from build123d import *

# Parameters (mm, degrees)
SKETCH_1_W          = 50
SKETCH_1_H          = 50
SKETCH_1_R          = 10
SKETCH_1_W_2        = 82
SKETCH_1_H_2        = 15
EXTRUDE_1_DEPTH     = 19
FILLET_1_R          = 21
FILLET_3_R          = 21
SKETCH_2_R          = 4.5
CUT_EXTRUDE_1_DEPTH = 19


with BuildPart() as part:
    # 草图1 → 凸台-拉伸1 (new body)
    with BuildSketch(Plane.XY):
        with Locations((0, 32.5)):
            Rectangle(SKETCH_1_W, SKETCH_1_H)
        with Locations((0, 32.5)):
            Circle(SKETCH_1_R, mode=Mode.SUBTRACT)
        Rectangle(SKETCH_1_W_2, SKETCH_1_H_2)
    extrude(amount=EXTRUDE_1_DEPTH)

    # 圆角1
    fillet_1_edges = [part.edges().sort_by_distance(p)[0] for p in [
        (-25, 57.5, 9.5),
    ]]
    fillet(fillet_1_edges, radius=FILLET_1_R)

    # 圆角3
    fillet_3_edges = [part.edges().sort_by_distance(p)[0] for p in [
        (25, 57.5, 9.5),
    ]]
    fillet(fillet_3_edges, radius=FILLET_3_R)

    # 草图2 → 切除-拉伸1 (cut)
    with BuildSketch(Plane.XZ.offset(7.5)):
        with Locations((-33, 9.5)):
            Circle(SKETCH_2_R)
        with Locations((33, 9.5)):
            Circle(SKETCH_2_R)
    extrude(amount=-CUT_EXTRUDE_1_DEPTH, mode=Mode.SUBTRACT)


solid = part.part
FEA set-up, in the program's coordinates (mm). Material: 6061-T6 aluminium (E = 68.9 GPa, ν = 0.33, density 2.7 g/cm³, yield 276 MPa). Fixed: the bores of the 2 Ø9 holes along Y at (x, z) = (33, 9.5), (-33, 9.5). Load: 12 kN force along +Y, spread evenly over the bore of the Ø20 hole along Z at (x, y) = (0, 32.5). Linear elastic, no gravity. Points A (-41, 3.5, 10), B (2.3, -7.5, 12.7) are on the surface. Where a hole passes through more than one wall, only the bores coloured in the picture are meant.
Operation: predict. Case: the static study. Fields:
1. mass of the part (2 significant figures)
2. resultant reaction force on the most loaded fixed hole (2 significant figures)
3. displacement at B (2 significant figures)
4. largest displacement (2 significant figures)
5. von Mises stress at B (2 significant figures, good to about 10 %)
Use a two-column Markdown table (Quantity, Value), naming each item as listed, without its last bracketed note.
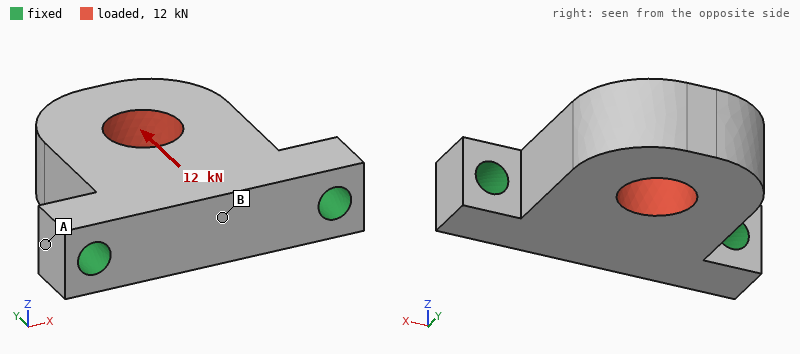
| Quantity | Value |
|---|---|
| mass of the part | 160 g |
| resultant reaction force on the most loaded fixed hole | 6.4 kN |
| displacement at B | 16 µm |
| largest displacement | 23 µm |
| von Mises stress at B | 15 MPa |
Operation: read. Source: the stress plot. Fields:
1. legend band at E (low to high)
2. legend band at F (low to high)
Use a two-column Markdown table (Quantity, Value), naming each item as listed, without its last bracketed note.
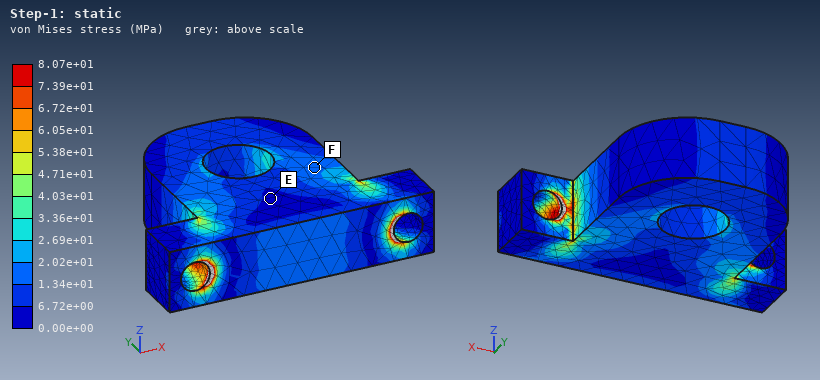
| Quantity | Value |
|---|---|
| legend band at E | 0.00e+00 to 6.72e+00 MPa |
| legend band at F | 1.34e+01 to 2.02e+01 MPa |
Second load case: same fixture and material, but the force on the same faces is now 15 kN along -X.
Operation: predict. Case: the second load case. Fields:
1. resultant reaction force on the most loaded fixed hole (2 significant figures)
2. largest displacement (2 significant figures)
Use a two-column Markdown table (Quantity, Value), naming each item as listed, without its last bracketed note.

| Quantity | Value |
|---|---|
| resultant reaction force on the most loaded fixed hole | 11 kN |
| largest displacement | 84 µm |
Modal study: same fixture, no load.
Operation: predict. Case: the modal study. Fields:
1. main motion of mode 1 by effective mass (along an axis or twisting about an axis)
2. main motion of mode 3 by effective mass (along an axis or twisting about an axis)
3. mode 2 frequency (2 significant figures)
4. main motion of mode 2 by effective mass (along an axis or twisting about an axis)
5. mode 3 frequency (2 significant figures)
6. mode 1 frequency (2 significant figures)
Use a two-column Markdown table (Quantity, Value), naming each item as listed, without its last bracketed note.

| Quantity | Value |
|---|---|
| main motion of mode 1 by effective mass | along Z |
| main motion of mode 3 by effective mass | twisting about Y |
| mode 2 frequency | 7800 Hz |
| main motion of mode 2 by effective mass | along X |
| mode 3 frequency | 9400 Hz |
| mode 1 frequency | 2900 Hz |
